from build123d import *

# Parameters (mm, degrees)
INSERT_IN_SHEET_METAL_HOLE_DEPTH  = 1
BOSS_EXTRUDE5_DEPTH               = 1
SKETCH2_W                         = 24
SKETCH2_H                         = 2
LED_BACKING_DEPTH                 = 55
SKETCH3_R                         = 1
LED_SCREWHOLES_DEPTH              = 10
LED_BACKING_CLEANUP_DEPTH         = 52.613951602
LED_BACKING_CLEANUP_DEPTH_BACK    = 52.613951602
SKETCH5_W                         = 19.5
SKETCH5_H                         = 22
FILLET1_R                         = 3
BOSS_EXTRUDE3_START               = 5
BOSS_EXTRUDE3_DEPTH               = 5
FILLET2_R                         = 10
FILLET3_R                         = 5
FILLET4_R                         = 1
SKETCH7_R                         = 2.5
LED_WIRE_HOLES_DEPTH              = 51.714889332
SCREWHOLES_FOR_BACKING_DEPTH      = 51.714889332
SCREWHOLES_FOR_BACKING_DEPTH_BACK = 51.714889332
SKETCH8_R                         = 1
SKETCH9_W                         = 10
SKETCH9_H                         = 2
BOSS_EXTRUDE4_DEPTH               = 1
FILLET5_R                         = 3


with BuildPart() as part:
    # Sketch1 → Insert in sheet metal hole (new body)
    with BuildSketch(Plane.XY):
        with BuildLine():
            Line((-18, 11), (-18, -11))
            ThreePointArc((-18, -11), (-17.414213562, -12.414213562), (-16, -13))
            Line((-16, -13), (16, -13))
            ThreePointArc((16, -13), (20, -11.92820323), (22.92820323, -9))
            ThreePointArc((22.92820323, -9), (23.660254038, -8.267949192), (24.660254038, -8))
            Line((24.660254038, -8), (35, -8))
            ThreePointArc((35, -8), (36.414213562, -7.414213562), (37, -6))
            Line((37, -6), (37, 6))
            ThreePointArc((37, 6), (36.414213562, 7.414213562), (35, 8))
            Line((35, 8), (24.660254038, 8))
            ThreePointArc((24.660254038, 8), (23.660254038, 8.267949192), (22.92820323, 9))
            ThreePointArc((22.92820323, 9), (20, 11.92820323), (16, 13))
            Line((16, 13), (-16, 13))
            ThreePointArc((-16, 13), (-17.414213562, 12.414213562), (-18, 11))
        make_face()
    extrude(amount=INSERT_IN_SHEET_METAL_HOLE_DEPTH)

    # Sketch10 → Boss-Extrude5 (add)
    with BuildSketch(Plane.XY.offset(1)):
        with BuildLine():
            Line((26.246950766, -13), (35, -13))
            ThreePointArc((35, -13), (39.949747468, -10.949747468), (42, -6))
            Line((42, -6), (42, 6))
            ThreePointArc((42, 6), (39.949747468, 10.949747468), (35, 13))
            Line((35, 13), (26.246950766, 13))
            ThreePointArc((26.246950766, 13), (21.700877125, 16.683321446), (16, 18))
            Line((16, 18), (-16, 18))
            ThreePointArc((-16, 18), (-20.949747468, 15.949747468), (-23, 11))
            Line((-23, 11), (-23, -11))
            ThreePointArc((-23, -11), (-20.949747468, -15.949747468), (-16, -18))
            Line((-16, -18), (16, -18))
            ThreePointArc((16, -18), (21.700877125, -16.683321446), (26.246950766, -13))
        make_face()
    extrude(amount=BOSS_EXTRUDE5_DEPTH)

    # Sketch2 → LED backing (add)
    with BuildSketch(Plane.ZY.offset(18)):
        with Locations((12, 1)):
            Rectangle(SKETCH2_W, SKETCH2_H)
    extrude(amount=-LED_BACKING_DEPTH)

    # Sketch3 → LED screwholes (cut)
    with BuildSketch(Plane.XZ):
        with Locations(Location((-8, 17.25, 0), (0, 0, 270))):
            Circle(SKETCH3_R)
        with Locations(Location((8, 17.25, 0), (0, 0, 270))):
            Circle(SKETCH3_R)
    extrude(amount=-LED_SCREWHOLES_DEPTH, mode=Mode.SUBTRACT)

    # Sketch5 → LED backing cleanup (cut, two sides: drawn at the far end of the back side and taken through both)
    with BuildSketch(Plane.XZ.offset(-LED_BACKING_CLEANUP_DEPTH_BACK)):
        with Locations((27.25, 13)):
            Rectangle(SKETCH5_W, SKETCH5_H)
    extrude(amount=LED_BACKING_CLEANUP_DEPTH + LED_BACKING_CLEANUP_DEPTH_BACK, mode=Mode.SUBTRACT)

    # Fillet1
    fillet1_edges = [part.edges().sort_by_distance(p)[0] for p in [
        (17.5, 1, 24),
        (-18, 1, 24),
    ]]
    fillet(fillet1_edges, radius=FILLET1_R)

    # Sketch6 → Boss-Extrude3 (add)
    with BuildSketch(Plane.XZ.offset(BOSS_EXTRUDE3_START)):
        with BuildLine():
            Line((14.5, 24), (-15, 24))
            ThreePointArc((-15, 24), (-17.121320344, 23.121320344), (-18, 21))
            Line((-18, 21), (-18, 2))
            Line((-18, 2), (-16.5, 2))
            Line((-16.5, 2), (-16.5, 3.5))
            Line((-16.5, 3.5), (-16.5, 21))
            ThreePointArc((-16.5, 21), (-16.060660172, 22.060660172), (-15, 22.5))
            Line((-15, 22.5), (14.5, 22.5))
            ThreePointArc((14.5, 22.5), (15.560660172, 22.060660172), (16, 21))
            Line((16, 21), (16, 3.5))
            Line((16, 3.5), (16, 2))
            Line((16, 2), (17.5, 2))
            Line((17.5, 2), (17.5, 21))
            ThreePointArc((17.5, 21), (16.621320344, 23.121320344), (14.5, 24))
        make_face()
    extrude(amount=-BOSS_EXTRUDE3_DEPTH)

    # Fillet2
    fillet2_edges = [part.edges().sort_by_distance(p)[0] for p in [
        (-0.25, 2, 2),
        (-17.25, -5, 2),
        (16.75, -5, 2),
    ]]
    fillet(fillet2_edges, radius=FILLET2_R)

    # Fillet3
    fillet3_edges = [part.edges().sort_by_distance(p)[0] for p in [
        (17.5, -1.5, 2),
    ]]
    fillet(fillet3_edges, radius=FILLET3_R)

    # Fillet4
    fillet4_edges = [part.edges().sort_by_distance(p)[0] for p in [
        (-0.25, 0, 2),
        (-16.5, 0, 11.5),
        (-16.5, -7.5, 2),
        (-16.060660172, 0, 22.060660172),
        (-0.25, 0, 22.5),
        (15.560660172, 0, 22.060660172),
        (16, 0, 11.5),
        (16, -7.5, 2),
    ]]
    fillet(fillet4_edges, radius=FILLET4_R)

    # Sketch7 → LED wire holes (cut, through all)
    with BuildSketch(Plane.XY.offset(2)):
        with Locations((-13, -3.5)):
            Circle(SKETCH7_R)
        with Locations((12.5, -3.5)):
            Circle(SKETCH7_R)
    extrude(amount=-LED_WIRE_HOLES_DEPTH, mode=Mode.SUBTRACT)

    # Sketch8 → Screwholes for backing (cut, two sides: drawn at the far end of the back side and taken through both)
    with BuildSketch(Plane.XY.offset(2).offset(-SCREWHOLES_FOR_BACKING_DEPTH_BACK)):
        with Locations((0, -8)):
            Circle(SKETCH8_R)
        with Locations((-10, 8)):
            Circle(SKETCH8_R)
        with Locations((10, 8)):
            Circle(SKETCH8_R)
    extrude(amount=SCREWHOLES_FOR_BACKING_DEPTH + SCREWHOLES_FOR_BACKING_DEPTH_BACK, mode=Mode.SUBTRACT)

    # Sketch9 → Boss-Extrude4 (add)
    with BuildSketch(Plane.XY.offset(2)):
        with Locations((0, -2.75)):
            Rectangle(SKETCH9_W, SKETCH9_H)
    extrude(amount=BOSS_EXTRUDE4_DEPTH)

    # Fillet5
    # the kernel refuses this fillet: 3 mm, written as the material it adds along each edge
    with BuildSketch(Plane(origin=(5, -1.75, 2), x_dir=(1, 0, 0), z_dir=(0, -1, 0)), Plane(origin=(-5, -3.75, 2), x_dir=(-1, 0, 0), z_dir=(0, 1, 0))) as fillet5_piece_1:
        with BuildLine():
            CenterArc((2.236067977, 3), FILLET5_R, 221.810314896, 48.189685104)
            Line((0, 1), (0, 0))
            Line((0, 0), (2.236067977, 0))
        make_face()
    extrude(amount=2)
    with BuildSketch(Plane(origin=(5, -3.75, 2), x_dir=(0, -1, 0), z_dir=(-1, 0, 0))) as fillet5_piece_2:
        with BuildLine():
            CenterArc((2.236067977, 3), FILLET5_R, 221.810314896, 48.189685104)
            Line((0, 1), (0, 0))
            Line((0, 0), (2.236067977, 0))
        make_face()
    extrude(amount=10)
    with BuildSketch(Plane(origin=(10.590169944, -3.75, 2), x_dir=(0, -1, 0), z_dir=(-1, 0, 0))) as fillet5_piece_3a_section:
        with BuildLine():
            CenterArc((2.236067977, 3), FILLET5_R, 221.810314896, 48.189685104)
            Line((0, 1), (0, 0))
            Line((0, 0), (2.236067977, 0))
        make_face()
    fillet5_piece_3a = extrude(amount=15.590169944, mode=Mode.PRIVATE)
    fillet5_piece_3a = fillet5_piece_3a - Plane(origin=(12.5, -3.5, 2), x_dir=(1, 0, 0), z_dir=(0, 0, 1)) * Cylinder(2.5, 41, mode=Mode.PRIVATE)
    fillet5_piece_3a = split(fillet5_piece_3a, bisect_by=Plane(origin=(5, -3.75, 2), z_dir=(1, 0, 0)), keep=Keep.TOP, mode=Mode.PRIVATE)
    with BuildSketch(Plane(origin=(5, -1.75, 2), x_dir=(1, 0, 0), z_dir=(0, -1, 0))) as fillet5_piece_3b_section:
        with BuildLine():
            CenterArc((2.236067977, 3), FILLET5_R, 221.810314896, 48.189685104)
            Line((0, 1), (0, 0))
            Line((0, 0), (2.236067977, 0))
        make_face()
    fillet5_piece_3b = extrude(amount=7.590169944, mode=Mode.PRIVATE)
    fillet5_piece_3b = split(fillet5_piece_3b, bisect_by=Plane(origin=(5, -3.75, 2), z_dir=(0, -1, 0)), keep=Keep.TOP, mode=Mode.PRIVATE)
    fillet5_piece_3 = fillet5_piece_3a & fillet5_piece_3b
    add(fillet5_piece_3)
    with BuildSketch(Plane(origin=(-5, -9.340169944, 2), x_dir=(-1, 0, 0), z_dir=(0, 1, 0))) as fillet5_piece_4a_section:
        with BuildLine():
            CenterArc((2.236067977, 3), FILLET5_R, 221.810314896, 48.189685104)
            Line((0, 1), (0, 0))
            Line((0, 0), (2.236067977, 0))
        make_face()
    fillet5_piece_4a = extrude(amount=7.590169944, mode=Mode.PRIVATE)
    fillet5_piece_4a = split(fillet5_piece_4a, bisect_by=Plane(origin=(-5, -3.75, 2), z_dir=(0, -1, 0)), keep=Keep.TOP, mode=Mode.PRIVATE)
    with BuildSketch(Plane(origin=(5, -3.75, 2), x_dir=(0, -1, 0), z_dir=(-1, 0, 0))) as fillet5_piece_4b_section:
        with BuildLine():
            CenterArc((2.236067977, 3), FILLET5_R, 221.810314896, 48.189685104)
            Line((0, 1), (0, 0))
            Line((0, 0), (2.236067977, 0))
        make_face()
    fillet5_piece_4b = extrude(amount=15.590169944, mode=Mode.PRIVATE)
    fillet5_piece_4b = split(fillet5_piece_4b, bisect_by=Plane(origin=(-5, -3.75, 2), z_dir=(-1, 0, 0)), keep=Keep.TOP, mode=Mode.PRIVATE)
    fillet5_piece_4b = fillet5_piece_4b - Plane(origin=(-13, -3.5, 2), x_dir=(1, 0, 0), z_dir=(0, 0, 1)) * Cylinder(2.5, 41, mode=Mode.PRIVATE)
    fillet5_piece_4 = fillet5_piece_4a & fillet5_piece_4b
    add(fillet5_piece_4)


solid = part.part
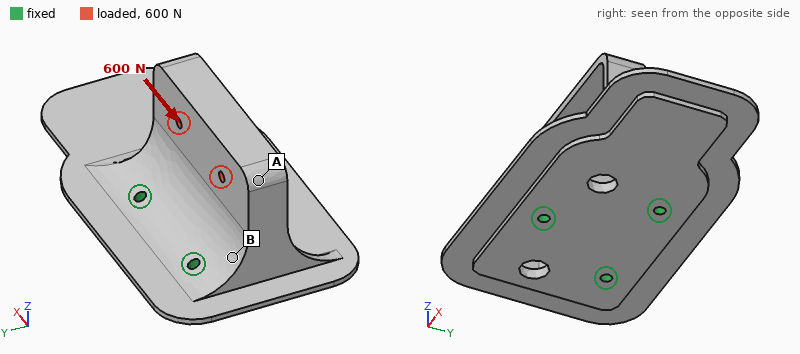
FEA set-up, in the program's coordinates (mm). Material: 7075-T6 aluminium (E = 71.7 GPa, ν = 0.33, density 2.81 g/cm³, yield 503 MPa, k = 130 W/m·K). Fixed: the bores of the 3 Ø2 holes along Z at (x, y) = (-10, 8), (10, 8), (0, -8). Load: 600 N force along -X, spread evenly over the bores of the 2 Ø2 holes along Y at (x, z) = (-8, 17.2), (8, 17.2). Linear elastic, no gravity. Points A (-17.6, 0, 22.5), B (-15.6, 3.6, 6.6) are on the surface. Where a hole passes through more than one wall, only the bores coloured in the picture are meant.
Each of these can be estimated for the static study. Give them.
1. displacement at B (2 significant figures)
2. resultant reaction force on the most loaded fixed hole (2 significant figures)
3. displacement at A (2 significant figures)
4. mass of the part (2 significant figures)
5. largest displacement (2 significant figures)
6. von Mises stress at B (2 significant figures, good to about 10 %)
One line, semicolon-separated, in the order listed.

13 µm; 520 N; 34 µm; 18 g; 53 µm; 9.6 MPa
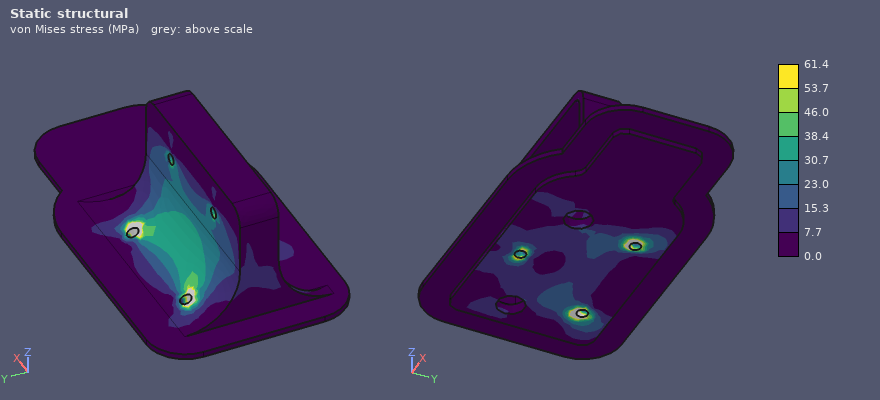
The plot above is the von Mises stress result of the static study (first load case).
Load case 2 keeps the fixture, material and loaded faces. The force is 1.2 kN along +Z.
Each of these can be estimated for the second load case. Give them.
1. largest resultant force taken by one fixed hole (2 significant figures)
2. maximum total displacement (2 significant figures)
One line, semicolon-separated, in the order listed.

440 N; 58 µm
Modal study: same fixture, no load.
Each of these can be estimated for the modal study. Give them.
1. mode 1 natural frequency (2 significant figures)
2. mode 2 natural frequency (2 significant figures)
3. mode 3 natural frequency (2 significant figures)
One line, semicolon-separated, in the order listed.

3300 Hz; 4900 Hz; 5900 Hz
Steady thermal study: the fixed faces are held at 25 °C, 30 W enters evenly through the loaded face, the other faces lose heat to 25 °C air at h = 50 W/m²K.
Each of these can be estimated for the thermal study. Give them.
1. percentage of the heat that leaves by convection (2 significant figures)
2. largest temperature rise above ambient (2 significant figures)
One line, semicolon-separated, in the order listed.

16 %; 53 K
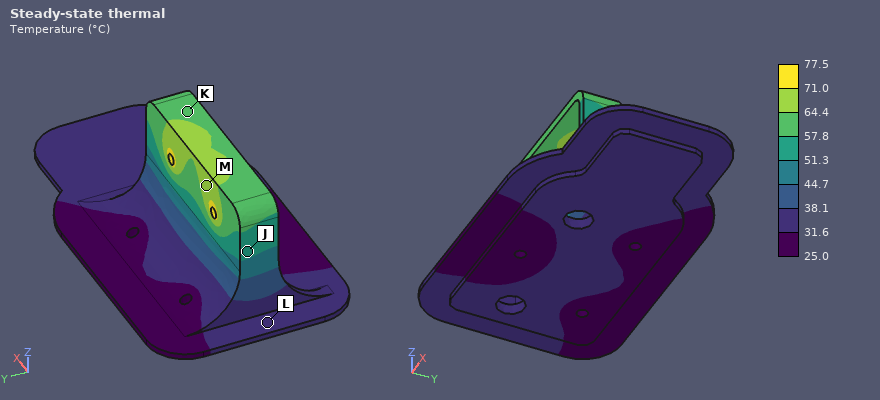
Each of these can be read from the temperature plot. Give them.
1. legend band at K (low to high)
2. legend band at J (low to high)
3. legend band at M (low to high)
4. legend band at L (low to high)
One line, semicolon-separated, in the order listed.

57.8 to 64.4 °C; 51.3 to 57.8 °C; 64.4 to 71.0 °C; 31.6 to 38.1 °C
